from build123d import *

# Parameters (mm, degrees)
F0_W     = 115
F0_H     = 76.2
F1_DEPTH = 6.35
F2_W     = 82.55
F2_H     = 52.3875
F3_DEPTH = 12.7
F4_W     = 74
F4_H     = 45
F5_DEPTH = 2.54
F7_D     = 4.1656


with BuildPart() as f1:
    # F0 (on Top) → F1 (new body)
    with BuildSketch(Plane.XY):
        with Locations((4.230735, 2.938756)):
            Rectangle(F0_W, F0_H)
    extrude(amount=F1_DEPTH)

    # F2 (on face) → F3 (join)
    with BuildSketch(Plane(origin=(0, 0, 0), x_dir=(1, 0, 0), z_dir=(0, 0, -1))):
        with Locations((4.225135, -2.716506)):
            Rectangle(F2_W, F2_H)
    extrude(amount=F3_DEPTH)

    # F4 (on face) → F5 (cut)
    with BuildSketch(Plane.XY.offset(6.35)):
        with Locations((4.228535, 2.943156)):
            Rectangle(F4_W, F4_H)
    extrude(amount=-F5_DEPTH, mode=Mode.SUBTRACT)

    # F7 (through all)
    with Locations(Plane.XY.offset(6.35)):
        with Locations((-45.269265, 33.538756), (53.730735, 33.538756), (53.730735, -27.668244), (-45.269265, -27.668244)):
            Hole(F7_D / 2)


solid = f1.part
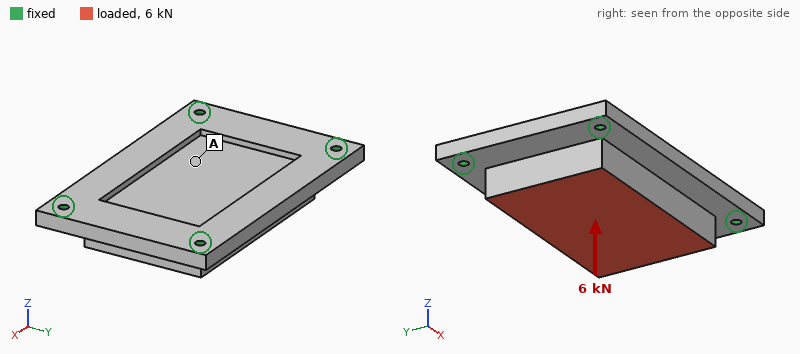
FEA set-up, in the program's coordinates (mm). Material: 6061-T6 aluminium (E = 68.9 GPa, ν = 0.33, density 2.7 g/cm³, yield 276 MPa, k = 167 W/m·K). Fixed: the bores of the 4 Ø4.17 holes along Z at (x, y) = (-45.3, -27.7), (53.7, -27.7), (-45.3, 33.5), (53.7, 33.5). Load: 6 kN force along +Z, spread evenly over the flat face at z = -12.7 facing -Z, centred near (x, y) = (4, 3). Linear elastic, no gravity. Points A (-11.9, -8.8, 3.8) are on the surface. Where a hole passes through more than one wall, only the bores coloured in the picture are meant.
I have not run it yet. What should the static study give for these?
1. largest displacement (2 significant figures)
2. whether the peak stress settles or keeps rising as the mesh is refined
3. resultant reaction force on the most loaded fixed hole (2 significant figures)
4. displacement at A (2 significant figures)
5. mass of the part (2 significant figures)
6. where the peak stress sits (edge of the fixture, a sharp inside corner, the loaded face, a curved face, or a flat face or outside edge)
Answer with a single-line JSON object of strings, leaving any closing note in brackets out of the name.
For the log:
{"largest displacement": "48 µm", "whether the peak stress settles or keeps rising as the mesh is refined": "keeps rising", "resultant reaction force on the most loaded fixed hole": "2.1 kN", "displacement at A": "42 µm", "mass of the part": "270 g", "where the peak stress sits": "edge of the fixture"}
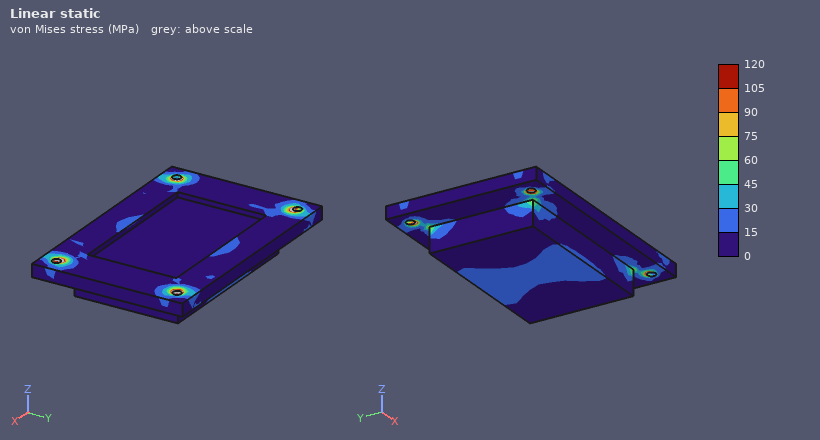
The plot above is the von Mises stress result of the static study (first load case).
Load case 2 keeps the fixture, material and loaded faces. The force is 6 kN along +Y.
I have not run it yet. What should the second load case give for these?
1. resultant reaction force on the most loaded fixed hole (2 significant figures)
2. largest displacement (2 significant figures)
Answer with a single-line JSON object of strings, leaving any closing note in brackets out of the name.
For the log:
{"resultant reaction force on the most loaded fixed hole": "2.0 kN", "largest displacement": "26 µm"}
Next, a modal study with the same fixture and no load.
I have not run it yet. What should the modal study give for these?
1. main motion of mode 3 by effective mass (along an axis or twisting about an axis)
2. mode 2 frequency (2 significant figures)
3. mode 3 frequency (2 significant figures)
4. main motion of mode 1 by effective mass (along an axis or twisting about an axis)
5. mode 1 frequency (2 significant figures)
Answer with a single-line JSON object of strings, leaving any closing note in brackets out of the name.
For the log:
{"main motion of mode 3 by effective mass": "twisting about Y", "mode 2 frequency": "5900 Hz", "mode 3 frequency": "7800 Hz", "main motion of mode 1 by effective mass": "along Z", "mode 1 frequency": "4000 Hz"}
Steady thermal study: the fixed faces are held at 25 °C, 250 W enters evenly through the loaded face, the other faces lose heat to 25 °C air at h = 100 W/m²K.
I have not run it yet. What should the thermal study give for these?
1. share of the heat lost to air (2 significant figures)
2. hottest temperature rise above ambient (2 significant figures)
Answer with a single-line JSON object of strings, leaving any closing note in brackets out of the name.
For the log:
{"share of the heat lost to air": "23 %", "hottest temperature rise above ambient": "47 K"}
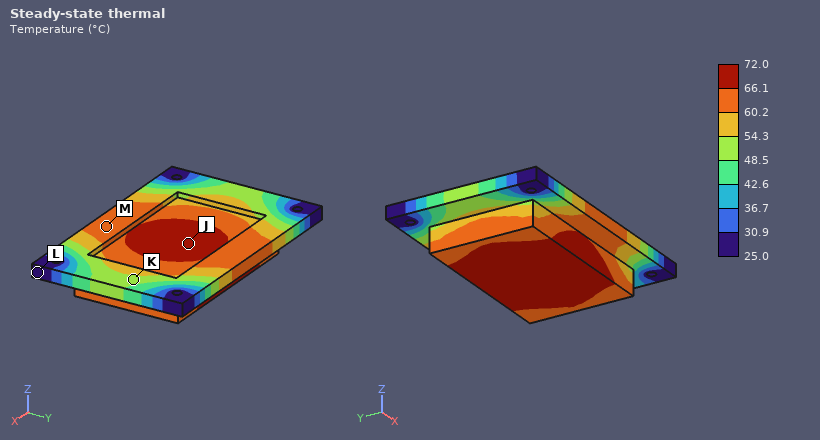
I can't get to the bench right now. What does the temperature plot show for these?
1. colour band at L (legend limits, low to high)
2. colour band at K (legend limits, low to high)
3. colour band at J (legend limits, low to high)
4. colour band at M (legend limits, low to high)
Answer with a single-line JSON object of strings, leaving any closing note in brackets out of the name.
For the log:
{"colour band at L": "25.0 to 30.9 °C", "colour band at K": "48.5 to 54.3 °C", "colour band at J": "66.1 to 72.0 °C", "colour band at M": "60.2 to 66.1 °C"}
